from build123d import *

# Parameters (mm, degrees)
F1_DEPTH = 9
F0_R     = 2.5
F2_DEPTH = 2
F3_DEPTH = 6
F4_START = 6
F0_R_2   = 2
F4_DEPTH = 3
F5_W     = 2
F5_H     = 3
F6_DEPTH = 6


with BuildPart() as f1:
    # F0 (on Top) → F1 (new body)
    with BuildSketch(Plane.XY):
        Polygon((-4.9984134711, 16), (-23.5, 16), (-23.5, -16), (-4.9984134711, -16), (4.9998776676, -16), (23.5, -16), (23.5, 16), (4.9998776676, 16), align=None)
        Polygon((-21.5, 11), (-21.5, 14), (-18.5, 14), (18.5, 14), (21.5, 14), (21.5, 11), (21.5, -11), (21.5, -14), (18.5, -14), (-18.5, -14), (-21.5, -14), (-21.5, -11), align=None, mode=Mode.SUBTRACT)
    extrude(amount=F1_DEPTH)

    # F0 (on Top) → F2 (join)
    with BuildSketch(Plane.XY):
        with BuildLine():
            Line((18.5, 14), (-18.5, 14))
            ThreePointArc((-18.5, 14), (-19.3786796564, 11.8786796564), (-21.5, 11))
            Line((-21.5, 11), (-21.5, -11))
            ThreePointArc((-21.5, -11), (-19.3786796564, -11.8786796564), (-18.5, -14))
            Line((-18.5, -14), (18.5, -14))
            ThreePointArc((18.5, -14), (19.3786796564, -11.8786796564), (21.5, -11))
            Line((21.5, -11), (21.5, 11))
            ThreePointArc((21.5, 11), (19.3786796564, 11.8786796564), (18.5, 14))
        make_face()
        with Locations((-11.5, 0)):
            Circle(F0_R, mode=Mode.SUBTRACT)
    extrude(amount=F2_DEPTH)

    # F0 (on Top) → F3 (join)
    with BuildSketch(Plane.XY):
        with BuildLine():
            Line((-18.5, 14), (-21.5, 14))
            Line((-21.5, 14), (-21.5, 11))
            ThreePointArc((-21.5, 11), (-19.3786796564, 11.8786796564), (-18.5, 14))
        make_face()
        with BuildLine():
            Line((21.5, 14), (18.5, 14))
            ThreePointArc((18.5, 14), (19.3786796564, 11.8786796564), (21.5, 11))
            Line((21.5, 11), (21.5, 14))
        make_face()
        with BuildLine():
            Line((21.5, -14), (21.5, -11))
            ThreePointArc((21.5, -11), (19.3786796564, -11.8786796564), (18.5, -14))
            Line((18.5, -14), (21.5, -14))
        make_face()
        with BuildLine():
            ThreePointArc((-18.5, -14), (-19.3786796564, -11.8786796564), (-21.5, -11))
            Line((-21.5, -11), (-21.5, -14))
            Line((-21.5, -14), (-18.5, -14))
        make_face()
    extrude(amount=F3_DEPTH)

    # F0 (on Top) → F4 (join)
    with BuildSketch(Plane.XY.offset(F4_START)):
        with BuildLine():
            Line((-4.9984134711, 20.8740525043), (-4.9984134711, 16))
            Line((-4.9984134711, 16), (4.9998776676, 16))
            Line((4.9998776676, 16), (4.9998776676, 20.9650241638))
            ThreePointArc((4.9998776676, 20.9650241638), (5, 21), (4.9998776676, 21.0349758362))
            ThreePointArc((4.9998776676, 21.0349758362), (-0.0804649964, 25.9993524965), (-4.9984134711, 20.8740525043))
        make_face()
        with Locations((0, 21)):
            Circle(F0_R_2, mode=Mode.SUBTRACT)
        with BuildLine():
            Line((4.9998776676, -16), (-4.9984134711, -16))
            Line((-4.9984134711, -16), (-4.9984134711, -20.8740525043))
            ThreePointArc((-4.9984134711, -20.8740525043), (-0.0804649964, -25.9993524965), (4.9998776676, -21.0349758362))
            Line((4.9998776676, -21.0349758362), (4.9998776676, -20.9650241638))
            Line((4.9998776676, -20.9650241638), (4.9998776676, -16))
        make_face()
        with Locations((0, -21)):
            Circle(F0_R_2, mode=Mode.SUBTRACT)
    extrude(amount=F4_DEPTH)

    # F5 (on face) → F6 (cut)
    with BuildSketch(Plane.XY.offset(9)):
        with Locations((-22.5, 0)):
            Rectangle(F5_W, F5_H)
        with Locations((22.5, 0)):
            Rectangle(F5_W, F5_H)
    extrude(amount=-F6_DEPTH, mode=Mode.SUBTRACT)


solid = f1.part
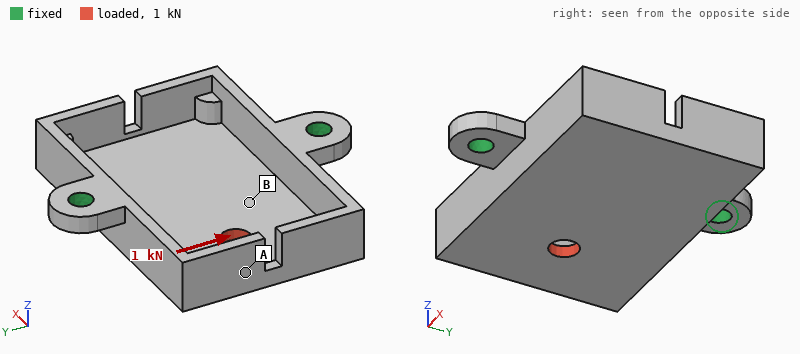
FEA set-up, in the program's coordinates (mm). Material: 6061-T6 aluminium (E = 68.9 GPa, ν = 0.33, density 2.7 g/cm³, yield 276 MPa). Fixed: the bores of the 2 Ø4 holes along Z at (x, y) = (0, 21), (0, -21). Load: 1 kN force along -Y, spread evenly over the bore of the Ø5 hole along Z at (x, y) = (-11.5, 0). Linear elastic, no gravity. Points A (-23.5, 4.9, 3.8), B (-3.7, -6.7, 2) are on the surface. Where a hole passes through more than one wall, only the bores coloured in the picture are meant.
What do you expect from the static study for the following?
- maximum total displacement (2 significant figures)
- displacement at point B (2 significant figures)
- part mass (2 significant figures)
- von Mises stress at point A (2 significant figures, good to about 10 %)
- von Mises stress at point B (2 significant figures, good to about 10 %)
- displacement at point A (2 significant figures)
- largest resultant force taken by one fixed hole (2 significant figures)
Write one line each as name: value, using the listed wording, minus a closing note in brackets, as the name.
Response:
maximum total displacement: 99 µm
displacement at point B: 44 µm
part mass: 15 g
von Mises stress at point A: 16 MPa
von Mises stress at point B: 44 MPa
displacement at point A: 71 µm
largest resultant force taken by one fixed hole: 600 N
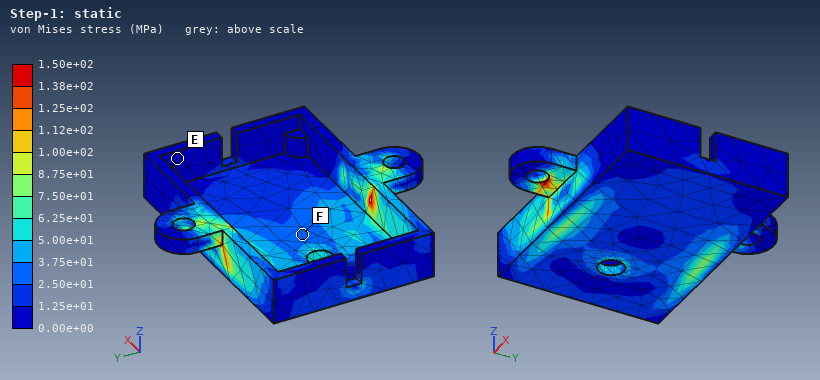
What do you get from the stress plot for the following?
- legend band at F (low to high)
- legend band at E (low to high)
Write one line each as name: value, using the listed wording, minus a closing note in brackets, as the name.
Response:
legend band at F: 2.50e+01 to 3.75e+01 MPa
legend band at E: 0.00e+00 to 1.25e+01 MPa
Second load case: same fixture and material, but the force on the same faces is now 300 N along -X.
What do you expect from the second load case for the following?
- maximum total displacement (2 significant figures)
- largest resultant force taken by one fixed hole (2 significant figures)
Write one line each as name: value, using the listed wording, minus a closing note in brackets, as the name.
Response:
maximum total displacement: 49 µm
largest resultant force taken by one fixed hole: 150 N
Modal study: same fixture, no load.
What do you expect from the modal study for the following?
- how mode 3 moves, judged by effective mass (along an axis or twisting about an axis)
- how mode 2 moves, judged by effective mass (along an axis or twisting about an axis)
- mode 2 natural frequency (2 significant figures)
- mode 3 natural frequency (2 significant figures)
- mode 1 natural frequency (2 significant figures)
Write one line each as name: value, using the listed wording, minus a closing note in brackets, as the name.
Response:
how mode 3 moves, judged by effective mass: along Z
how mode 2 moves, judged by effective mass: twisting about Z
mode 2 natural frequency: 4600 Hz
mode 3 natural frequency: 6200 Hz
mode 1 natural frequency: 2600 Hz
